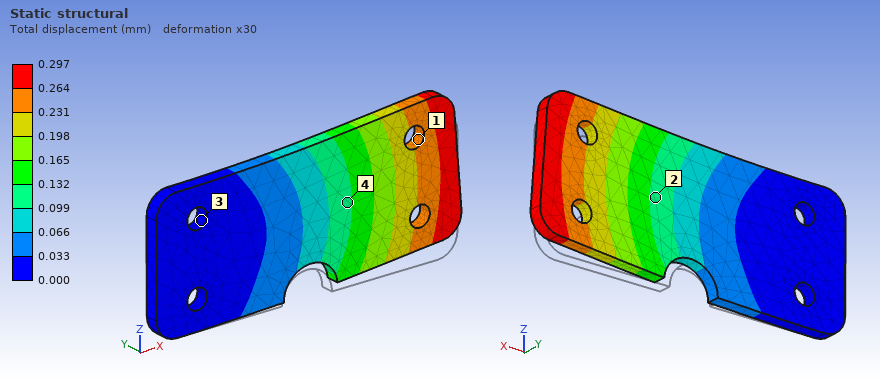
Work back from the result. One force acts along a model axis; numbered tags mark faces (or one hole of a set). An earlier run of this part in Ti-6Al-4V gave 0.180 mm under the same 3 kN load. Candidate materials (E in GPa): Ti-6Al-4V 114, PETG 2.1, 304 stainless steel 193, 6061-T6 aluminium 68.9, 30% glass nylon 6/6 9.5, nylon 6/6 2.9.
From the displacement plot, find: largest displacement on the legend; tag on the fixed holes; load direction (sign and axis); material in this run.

0.297 mm
3
+Z
6061-T6 aluminium
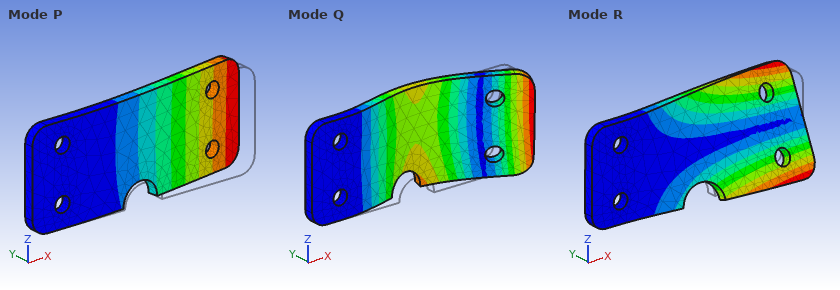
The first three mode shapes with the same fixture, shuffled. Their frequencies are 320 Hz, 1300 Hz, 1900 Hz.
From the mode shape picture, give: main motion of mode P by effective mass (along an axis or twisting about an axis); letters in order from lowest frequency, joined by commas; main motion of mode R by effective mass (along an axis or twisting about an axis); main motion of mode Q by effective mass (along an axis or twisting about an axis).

along Y
P, R, Q
twisting about X
along Y
